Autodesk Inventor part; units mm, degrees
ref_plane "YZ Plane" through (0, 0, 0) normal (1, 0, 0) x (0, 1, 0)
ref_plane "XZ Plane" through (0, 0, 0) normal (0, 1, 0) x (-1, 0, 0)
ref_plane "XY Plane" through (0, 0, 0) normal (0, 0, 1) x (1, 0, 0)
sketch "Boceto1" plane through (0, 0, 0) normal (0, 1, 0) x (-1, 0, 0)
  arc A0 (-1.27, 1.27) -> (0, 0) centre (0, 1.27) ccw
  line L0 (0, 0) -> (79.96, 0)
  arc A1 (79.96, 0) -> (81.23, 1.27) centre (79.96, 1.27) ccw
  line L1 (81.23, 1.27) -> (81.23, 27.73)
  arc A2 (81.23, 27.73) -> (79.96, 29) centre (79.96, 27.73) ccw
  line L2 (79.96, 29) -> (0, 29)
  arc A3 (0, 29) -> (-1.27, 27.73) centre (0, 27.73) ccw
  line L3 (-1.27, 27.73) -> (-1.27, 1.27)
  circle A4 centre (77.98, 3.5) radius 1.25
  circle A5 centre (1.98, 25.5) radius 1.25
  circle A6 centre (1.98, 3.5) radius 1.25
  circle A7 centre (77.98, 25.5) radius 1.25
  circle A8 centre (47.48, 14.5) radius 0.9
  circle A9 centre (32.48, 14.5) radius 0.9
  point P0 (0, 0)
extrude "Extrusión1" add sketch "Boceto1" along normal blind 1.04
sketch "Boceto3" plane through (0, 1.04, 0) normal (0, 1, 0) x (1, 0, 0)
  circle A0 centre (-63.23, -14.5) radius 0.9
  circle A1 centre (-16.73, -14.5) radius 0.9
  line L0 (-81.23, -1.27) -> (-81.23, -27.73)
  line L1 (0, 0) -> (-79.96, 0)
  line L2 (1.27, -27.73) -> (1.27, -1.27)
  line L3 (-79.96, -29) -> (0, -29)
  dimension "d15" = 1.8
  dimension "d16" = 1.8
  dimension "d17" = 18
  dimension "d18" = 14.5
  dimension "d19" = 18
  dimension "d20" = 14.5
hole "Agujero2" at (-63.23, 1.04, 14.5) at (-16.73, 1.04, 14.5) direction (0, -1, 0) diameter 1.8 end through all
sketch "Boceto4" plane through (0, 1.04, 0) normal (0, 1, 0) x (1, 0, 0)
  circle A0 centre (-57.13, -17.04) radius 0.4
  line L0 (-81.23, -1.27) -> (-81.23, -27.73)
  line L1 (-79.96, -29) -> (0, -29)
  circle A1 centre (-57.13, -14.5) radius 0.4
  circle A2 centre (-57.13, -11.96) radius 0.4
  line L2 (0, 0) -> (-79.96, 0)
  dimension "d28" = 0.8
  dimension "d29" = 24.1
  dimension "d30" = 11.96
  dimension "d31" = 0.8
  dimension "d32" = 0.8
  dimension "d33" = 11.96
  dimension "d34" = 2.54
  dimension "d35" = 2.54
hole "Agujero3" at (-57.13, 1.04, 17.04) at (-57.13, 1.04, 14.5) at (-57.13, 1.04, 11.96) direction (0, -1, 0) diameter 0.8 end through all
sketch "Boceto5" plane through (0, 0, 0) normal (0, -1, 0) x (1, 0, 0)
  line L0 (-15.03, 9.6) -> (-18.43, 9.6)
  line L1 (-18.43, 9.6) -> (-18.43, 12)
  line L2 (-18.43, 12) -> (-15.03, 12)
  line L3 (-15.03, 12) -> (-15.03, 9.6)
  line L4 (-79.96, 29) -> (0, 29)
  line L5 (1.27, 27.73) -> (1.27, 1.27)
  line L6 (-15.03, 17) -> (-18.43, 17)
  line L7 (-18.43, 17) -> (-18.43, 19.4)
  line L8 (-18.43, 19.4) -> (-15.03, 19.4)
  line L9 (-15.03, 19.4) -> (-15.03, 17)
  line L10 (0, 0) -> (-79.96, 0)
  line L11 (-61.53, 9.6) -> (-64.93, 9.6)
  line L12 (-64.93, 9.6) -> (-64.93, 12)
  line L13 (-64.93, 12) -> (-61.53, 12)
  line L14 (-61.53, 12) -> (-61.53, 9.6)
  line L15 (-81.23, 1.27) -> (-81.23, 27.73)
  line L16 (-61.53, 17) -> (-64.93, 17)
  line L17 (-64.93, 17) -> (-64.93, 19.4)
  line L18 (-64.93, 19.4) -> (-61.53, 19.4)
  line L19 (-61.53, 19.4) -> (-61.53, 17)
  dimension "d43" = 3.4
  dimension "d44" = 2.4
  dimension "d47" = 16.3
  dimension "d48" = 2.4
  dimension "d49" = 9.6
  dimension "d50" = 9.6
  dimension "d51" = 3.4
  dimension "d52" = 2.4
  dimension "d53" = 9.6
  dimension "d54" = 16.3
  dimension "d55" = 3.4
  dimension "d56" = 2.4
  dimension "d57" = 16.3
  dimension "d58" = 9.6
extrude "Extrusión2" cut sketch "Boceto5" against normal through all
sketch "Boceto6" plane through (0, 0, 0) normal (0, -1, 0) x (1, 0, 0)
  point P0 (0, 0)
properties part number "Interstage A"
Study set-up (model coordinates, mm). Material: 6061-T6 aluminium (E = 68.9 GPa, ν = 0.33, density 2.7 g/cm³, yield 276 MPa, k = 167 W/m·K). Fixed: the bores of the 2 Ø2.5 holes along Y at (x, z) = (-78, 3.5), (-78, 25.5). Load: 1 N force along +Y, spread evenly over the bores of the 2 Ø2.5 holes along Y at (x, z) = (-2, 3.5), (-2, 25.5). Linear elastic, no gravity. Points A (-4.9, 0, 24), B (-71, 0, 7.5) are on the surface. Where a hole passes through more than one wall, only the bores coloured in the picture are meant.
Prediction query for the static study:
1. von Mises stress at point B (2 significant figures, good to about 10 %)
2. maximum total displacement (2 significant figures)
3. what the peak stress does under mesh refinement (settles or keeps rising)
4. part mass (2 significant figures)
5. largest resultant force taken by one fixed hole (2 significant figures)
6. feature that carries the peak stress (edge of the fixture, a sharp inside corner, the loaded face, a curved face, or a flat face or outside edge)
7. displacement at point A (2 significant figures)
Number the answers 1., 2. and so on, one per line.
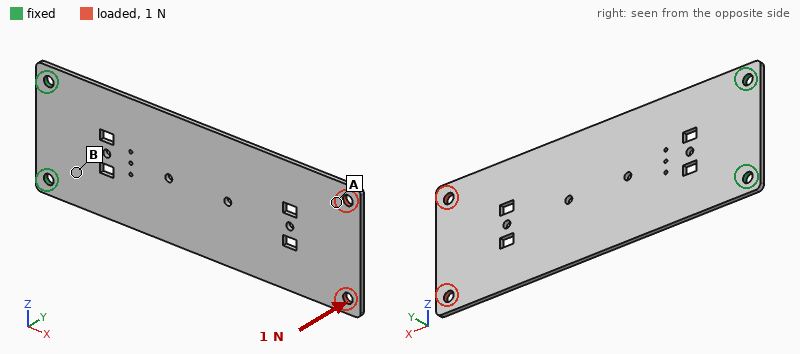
1. 12 MPa
2. 0.88 mm
3. keeps rising
4. 6.5 g
5. 0.50 N
6. edge of the fixture
7. 0.78 mm
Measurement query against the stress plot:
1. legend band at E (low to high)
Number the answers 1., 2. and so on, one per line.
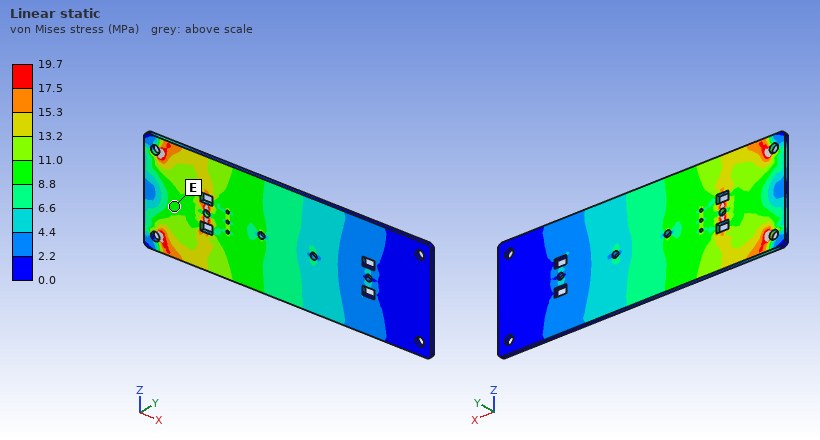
1. 8.8 to 11.0 MPa
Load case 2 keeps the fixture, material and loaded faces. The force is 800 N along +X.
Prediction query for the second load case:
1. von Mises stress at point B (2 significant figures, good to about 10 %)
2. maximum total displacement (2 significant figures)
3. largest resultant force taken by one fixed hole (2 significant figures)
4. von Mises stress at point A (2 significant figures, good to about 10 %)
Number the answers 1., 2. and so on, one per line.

1. 29 MPa
2. 39 µm
3. 410 N
4. 49 MPa
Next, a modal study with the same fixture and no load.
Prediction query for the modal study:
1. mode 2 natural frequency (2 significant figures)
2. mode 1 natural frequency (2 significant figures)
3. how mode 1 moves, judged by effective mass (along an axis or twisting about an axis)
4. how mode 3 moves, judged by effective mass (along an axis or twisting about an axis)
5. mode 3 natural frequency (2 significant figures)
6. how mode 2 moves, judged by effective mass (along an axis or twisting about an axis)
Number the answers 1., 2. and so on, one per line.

1. 770 Hz
2. 130 Hz
3. along Y
4. along Y
5. 850 Hz
6. twisting about X
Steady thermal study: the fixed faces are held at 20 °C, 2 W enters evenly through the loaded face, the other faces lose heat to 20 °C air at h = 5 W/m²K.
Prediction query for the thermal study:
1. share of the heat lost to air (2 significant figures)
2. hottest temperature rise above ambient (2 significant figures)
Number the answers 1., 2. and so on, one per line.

1. 18 %
2. 31 K
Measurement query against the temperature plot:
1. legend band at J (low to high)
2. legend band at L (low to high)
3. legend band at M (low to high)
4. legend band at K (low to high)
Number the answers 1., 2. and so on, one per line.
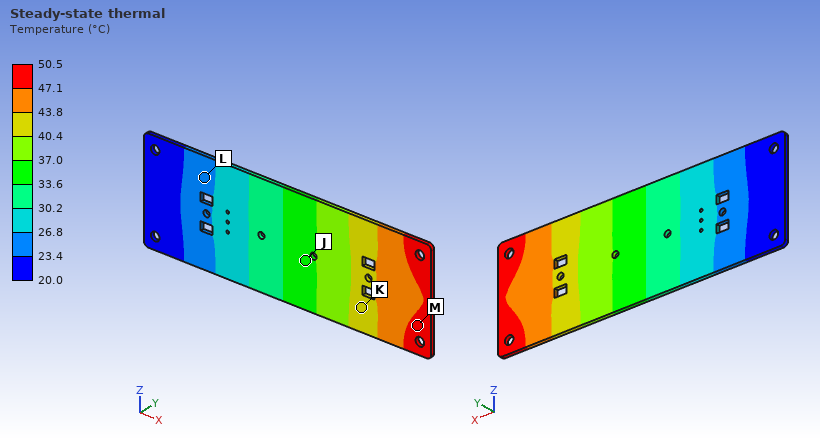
1. 33.6 to 37.0 °C
2. 23.4 to 26.8 °C
3. 47.1 to 50.5 °C
4. 40.4 to 43.8 °C
